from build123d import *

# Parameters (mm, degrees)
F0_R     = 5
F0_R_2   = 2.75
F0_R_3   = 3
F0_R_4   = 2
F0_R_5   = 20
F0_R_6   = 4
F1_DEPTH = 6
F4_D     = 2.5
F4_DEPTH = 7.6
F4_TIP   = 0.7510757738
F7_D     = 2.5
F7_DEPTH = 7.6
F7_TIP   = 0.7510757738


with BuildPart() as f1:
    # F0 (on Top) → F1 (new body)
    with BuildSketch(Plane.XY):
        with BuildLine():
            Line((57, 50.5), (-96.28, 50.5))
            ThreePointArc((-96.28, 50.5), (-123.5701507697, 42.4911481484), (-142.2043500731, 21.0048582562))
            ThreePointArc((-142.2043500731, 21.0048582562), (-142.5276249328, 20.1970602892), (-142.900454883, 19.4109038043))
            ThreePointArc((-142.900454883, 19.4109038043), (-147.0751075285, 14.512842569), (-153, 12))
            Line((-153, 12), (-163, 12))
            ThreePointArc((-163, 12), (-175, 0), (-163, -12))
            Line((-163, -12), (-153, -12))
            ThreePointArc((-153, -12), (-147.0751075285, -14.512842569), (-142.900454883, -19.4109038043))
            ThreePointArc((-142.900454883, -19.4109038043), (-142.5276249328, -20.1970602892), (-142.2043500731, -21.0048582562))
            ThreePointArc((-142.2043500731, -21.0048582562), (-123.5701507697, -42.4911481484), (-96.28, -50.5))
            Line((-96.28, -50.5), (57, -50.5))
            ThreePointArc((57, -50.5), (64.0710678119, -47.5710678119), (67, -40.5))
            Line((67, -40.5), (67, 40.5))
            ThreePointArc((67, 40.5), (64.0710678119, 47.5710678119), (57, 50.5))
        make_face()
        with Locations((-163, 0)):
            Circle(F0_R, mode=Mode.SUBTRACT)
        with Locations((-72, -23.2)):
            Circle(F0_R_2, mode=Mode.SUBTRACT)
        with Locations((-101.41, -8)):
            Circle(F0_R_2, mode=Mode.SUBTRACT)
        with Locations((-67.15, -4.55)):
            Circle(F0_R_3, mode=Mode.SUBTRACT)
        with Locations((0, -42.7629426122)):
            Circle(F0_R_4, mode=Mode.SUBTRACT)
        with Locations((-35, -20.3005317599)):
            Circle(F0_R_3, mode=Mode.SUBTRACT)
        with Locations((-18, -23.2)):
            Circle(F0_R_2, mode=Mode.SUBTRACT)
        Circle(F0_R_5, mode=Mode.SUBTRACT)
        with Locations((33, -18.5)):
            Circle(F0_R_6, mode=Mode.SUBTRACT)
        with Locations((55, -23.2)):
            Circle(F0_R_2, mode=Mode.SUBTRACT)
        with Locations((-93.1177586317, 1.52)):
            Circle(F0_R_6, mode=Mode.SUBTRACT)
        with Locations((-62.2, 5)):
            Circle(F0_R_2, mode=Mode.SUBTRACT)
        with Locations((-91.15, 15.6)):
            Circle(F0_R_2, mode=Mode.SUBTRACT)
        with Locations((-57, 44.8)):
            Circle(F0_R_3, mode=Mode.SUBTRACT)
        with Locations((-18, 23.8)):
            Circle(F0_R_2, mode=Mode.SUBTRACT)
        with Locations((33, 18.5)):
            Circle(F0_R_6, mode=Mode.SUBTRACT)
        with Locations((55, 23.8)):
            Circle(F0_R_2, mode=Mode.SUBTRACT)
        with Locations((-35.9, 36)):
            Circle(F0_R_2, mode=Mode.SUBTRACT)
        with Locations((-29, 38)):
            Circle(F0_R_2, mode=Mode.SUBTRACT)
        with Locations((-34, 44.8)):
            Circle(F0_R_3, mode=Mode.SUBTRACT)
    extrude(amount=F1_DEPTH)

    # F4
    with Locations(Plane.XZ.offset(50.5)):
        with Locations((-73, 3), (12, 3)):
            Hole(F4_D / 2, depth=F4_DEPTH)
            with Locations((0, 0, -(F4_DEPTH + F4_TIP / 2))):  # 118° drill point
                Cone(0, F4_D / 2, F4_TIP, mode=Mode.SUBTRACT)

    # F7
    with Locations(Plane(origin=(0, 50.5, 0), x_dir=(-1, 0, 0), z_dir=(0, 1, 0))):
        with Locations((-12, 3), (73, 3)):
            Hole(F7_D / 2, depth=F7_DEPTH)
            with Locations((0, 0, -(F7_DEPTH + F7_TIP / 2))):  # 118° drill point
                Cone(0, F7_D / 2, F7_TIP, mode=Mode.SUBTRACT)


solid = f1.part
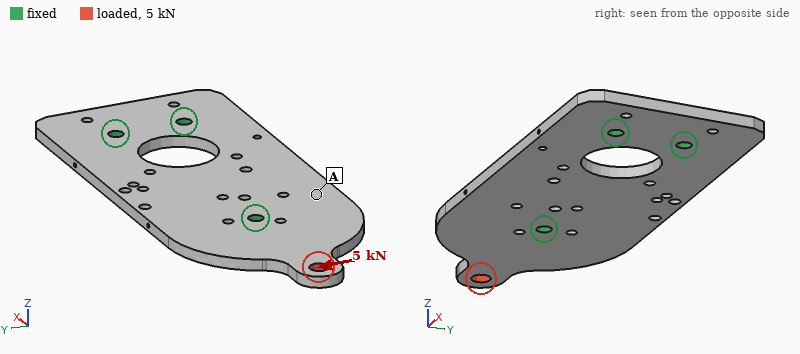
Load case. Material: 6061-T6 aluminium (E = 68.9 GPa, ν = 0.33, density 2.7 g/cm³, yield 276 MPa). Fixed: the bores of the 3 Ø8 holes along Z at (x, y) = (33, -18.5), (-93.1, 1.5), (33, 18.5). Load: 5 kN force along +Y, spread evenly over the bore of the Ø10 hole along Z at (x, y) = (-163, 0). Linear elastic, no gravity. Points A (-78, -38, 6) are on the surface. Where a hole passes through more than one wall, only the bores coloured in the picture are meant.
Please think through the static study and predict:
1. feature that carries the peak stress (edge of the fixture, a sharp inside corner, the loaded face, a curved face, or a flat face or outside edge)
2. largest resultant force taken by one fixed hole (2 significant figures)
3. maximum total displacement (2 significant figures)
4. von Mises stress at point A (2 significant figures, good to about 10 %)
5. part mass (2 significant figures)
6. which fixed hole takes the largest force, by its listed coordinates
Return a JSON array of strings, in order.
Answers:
["the loaded face", "7.1 kN", "0.23 mm", "25 MPa", "310 g", "(-93.1, 1.5)"]
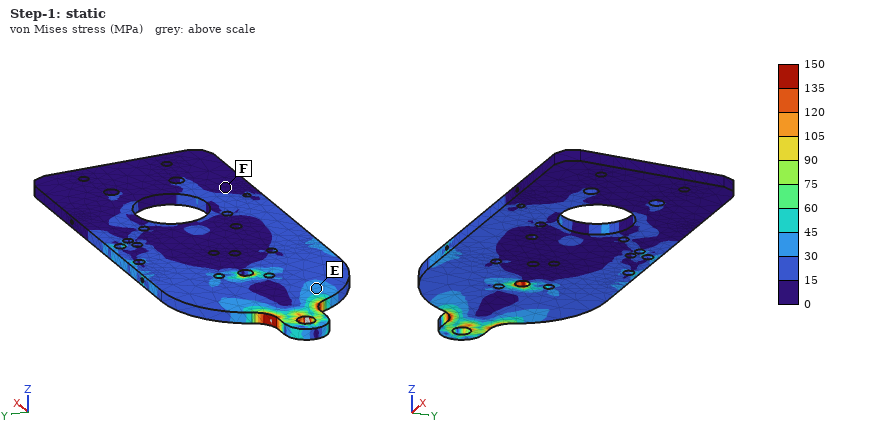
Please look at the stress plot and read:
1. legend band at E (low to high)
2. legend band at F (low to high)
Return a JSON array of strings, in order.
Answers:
["30 to 45 MPa", "0 to 15 MPa"]
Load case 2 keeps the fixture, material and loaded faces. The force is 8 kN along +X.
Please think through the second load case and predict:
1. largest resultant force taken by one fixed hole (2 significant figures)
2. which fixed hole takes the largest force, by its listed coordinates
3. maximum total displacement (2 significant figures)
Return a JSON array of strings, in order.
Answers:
["6.6 kN", "(-93.1, 1.5)", "54 µm"]
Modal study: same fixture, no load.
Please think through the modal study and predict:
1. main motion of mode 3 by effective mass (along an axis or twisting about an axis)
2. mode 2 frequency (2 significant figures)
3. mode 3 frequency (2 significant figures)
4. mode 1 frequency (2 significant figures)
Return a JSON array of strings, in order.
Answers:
["along Z", "1400 Hz", "1600 Hz", "1200 Hz"]
